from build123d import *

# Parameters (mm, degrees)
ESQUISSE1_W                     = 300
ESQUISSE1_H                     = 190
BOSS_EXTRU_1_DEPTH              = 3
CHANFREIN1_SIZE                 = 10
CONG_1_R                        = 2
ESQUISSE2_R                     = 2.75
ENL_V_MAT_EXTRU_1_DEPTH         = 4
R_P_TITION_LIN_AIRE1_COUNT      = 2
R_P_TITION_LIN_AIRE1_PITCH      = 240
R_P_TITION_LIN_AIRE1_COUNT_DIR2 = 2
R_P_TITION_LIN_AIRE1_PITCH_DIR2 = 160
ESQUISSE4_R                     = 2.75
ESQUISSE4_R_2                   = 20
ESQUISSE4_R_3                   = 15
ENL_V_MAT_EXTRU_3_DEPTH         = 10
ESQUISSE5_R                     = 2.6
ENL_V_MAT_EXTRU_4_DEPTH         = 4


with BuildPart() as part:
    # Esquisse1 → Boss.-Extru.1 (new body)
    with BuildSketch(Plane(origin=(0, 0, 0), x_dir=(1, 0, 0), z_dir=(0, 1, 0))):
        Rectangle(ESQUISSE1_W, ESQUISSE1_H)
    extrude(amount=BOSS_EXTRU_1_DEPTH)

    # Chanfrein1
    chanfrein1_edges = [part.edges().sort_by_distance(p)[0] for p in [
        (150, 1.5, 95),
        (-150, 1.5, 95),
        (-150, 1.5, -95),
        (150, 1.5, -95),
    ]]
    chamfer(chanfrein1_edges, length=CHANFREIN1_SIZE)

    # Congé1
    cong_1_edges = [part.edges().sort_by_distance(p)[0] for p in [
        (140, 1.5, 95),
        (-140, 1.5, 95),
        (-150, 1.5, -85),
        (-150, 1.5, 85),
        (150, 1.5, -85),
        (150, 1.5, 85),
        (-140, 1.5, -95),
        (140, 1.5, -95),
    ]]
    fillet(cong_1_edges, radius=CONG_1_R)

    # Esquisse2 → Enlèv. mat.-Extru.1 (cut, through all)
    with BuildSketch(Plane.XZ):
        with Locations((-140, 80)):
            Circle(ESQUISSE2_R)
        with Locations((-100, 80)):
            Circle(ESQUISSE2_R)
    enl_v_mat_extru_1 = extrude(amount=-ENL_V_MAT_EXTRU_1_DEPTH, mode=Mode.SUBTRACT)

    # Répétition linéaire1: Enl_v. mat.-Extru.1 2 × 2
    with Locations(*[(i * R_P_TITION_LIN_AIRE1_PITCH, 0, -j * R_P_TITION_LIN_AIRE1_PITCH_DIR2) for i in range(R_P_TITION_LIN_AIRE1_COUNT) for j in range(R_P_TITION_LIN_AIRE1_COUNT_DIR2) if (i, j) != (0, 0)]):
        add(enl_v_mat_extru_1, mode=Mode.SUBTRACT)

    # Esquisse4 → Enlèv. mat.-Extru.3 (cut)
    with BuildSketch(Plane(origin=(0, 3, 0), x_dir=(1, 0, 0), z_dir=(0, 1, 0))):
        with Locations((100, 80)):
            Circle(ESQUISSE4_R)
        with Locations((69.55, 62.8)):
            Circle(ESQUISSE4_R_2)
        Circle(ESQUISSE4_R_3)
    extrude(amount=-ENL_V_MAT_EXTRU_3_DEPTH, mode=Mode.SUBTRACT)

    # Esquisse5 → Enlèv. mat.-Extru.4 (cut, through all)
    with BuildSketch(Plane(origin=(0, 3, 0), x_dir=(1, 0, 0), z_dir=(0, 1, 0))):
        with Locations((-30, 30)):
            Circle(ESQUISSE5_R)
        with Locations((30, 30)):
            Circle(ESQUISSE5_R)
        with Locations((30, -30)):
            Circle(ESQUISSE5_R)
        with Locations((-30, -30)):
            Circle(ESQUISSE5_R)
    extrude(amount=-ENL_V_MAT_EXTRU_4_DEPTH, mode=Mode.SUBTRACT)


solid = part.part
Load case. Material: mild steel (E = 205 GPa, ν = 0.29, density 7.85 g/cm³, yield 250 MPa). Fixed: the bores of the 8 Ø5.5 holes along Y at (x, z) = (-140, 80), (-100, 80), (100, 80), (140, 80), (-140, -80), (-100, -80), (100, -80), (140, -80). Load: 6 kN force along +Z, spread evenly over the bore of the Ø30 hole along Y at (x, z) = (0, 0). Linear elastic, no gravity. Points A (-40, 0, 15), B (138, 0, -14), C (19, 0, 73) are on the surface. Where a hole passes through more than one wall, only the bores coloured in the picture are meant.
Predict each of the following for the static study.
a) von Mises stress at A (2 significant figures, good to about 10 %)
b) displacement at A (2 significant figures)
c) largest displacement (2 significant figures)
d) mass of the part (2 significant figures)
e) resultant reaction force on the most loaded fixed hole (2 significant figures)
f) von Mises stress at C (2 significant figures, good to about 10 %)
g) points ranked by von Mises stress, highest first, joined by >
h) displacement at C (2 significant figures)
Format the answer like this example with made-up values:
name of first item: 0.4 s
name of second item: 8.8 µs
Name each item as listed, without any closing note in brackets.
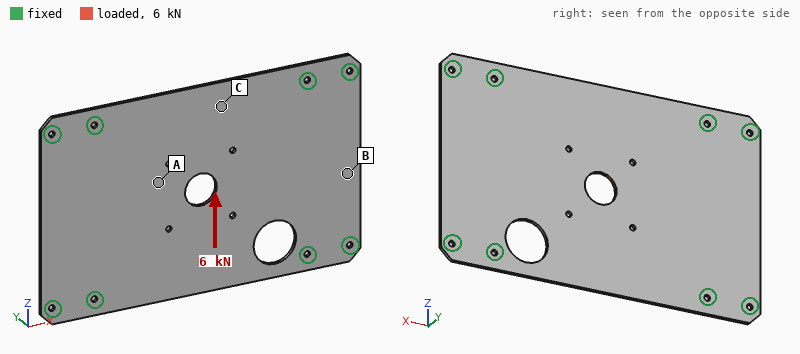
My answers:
von Mises stress at A: 13 MPa
displacement at A: 7.4 µm
largest displacement: 12 µm
mass of the part: 1.3 kg
resultant reaction force on the most loaded fixed hole: 1.6 kN
von Mises stress at C: 6.5 MPa
points ranked by von Mises stress, highest first, joined by >: A > C > B
displacement at C: 8.6 µm
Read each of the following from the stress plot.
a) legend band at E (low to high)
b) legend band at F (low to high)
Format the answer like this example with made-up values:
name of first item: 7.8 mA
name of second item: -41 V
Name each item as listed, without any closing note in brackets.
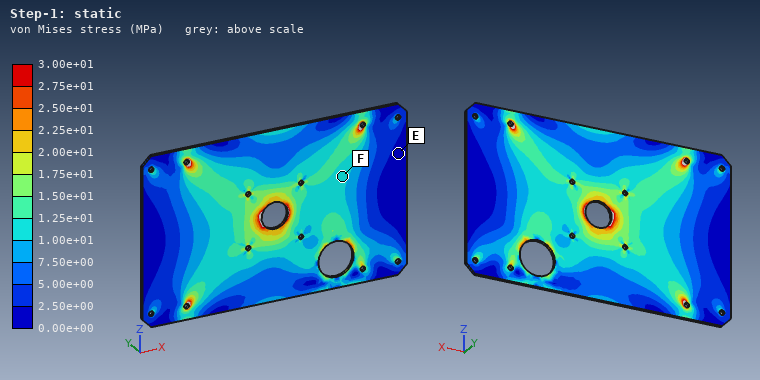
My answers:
legend band at E: 0.00e+00 to 2.50e+00 MPa
legend band at F: 1.00e+01 to 1.25e+01 MPa
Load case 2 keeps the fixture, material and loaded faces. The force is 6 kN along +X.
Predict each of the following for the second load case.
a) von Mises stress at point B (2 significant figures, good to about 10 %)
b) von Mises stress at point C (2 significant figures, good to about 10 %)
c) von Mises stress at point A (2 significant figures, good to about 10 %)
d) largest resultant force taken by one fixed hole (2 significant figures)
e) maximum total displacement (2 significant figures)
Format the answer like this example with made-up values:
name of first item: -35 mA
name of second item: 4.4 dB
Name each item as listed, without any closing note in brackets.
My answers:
von Mises stress at point B: 3.3 MPa
von Mises stress at point C: 2.8 MPa
von Mises stress at point A: 12 MPa
largest resultant force taken by one fixed hole: 1.2 kN
maximum total displacement: 8.3 µm
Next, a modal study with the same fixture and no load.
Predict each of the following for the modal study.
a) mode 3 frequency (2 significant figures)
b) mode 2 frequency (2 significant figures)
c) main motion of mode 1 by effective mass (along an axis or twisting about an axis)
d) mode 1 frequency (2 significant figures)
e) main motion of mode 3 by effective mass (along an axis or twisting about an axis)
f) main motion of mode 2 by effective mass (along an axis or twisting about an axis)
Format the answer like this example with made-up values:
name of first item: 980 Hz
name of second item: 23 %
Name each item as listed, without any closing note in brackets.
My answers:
mode 3 frequency: 600 Hz
mode 2 frequency: 460 Hz
main motion of mode 1 by effective mass: along Y
mode 1 frequency: 300 Hz
main motion of mode 3 by effective mass: twisting about Z
main motion of mode 2 by effective mass: twisting about X
